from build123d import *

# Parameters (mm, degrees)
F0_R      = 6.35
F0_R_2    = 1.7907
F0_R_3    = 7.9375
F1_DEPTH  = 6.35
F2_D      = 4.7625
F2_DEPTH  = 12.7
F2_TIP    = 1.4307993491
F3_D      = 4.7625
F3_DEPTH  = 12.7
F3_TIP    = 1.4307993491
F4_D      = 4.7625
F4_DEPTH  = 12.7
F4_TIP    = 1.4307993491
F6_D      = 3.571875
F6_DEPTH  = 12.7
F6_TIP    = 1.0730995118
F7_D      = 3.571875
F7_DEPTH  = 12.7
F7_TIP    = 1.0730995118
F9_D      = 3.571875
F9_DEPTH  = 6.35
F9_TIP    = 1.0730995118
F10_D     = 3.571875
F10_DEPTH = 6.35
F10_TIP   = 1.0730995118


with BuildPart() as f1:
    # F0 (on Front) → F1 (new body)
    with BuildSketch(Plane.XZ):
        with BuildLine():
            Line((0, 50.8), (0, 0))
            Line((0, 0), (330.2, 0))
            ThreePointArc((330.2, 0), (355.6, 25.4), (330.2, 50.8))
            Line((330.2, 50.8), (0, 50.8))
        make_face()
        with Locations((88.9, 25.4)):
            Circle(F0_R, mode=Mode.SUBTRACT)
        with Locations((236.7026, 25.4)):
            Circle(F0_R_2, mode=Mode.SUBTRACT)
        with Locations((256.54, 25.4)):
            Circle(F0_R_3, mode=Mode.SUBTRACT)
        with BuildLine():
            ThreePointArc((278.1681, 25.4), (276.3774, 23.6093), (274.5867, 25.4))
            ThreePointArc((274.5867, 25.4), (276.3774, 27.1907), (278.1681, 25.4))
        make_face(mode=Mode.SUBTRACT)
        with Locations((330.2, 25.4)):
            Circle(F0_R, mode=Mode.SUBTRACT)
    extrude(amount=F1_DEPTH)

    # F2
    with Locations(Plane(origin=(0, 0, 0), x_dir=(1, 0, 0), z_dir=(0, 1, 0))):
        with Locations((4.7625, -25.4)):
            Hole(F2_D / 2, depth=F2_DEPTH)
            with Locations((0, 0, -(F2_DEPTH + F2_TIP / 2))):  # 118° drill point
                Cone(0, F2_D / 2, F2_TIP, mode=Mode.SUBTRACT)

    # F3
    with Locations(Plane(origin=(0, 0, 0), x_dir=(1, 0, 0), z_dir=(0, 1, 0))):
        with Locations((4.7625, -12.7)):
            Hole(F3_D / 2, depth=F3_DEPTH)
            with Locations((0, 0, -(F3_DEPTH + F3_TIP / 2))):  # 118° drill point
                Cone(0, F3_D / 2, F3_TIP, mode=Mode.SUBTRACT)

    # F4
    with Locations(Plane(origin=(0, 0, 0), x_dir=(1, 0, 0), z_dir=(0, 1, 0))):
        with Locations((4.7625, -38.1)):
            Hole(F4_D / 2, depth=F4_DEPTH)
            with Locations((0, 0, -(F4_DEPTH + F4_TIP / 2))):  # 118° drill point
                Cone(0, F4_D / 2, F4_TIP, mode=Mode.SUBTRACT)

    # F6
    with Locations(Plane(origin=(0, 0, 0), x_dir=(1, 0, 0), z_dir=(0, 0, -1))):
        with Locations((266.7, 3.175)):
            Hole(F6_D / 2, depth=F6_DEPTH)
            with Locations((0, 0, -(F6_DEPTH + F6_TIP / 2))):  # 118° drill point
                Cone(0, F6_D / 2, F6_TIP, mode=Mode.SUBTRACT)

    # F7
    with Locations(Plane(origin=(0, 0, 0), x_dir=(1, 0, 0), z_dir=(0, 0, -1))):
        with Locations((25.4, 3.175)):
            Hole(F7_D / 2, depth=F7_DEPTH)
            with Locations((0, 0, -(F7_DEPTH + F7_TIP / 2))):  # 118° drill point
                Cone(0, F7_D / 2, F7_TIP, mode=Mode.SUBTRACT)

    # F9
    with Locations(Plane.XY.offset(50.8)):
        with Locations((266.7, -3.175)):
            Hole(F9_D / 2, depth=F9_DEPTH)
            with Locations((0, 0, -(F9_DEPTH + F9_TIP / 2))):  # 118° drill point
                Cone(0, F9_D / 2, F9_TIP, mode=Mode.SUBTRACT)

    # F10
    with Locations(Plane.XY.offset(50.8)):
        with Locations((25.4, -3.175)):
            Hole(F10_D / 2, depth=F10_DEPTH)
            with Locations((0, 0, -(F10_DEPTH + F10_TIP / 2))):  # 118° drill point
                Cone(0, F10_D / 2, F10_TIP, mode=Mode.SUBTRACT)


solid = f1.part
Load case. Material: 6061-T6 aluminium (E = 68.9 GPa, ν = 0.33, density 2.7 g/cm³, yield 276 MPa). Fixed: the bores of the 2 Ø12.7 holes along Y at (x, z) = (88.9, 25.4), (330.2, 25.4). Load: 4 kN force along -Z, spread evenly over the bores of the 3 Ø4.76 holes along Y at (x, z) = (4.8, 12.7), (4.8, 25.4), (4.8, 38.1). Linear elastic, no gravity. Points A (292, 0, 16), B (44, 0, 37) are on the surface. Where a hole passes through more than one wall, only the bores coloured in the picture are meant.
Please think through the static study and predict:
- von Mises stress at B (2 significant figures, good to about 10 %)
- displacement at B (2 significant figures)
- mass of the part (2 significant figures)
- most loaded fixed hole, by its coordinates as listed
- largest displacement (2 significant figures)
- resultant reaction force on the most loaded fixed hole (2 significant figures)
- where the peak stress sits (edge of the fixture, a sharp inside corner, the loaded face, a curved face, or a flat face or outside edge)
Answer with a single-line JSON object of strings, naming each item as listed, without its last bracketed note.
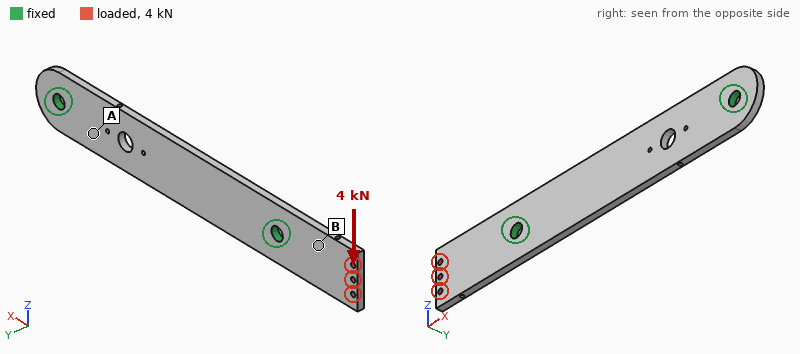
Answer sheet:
{"von Mises stress at B": "37 MPa", "displacement at B": "0.18 mm", "mass of the part": "290 g", "most loaded fixed hole, by its coordinates as listed": "(88.9, 25.4)", "largest displacement": "0.43 mm", "resultant reaction force on the most loaded fixed hole": "4.7 kN", "where the peak stress sits": "edge of the fixture"}
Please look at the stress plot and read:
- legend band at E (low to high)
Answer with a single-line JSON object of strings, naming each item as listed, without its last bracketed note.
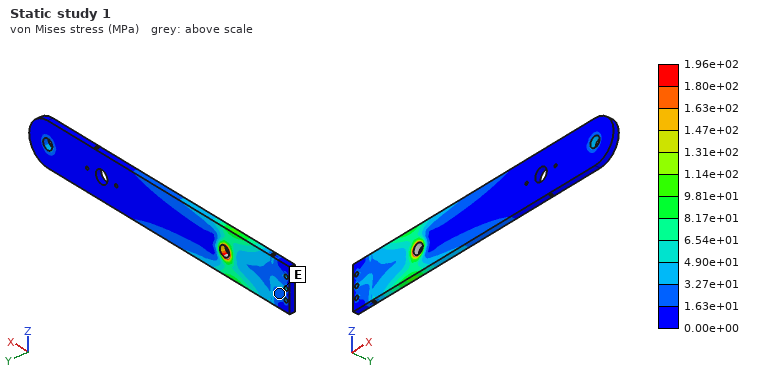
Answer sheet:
{"legend band at E": "1.63e+01 to 3.27e+01 MPa"}
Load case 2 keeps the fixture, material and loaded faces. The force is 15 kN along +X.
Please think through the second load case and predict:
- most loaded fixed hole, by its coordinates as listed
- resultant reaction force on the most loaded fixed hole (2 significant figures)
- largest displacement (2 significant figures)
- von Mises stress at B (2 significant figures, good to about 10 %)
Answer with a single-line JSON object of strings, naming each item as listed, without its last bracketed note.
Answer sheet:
{"most loaded fixed hole, by its coordinates as listed": "(88.9, 25.4)", "resultant reaction force on the most loaded fixed hole": "14 kN", "largest displacement": "76 µm", "von Mises stress at B": "49 MPa"}
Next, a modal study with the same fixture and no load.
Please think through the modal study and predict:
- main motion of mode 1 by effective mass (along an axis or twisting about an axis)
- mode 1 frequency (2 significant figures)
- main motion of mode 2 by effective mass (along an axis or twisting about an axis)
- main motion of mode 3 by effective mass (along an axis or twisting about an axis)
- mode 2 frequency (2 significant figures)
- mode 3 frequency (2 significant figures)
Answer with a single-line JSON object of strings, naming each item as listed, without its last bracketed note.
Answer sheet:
{"main motion of mode 1 by effective mass": "along Y", "mode 1 frequency": "600 Hz", "main motion of mode 2 by effective mass": "along Y", "main motion of mode 3 by effective mass": "twisting about X", "mode 2 frequency": "730 Hz", "mode 3 frequency": "1600 Hz"}
